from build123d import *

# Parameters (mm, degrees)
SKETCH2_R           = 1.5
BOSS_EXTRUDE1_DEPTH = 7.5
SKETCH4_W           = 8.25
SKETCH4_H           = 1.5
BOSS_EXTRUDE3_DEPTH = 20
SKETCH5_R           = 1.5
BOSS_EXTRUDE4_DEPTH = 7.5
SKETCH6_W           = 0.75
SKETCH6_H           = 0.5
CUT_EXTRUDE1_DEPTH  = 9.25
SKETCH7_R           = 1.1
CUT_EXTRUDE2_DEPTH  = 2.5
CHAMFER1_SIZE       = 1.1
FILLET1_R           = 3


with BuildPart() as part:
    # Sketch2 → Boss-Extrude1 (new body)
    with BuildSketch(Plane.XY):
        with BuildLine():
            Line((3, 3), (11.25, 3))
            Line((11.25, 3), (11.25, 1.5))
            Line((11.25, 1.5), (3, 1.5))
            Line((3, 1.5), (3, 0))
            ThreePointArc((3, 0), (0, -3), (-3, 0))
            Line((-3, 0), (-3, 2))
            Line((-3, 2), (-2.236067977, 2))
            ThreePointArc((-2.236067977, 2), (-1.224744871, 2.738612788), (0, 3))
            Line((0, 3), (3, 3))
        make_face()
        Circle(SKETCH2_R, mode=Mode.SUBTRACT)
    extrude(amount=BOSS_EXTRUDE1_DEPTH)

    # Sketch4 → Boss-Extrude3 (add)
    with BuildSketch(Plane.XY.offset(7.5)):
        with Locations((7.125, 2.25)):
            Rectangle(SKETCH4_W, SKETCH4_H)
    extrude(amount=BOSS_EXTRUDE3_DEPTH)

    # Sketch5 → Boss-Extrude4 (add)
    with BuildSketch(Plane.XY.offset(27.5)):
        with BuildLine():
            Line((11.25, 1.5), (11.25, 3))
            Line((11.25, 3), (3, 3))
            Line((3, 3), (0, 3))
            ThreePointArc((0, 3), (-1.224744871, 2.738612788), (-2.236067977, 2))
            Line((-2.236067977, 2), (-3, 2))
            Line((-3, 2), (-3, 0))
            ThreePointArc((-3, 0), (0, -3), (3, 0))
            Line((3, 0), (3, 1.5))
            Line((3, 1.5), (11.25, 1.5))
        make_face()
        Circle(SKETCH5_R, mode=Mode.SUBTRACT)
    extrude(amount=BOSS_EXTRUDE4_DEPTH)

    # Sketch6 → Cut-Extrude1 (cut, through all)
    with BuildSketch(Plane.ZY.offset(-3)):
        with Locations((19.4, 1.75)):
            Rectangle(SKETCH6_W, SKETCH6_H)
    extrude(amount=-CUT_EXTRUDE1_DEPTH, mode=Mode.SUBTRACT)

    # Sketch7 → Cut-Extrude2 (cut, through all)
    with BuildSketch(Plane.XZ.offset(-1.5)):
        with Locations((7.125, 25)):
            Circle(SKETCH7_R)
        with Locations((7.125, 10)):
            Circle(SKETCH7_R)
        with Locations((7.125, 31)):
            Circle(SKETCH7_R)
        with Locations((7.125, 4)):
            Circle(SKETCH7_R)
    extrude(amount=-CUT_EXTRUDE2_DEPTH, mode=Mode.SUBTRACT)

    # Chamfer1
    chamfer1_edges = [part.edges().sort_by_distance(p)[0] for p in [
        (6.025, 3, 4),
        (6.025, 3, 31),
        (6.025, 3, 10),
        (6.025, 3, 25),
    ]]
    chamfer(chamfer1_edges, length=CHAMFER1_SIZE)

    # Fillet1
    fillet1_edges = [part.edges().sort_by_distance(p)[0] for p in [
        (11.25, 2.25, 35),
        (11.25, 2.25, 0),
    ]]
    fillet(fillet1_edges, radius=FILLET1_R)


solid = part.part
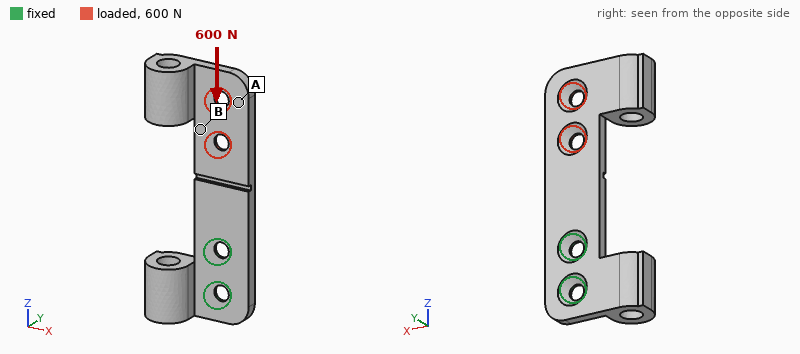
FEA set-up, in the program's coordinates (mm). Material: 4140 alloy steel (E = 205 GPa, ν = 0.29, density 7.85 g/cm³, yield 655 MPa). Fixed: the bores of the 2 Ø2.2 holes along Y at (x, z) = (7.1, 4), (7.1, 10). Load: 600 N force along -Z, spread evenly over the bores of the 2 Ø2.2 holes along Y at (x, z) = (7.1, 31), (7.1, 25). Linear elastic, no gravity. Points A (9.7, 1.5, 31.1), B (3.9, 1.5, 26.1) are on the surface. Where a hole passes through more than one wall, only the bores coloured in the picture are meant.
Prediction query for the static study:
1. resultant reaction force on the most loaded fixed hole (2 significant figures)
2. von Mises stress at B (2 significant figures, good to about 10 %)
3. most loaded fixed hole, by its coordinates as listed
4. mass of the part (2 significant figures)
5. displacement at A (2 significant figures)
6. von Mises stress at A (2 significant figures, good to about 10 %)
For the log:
500 N
130 MPa
(7.1, 10)
5.8 g
0.19 mm
43 MPa
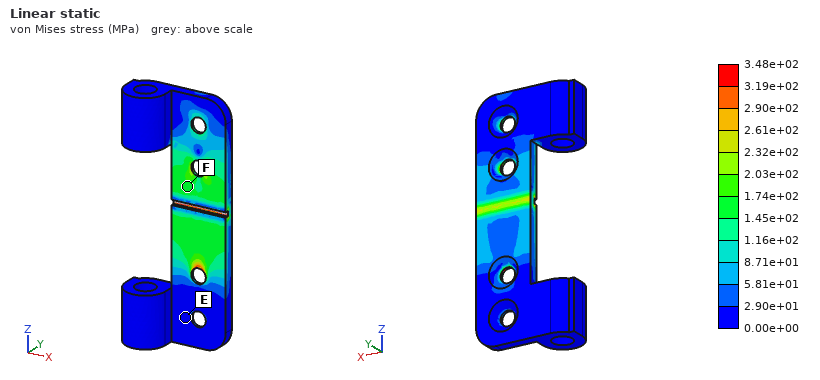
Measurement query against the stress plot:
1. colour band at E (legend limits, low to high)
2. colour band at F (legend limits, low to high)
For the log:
0.00e+00 to 2.90e+01 MPa
1.45e+02 to 1.74e+02 MPa
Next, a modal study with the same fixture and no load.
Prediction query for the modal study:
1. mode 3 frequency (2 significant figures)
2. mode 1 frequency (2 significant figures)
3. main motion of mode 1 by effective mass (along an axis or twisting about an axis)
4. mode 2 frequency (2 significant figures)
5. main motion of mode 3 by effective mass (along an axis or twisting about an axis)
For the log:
5200 Hz
1000 Hz
along Y
3600 Hz
along X
